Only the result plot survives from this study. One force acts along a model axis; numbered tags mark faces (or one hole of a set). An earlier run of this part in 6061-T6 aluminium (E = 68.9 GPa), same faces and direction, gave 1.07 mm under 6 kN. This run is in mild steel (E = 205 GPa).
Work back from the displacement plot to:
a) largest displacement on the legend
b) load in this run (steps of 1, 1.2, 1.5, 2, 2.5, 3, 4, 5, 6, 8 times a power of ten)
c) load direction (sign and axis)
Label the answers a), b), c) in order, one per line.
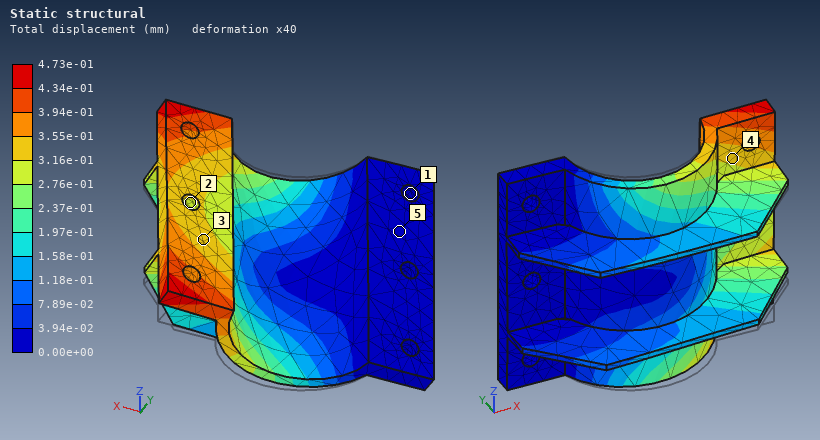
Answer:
a) 4.73e-01 mm
b) 8 kN
c) +Z
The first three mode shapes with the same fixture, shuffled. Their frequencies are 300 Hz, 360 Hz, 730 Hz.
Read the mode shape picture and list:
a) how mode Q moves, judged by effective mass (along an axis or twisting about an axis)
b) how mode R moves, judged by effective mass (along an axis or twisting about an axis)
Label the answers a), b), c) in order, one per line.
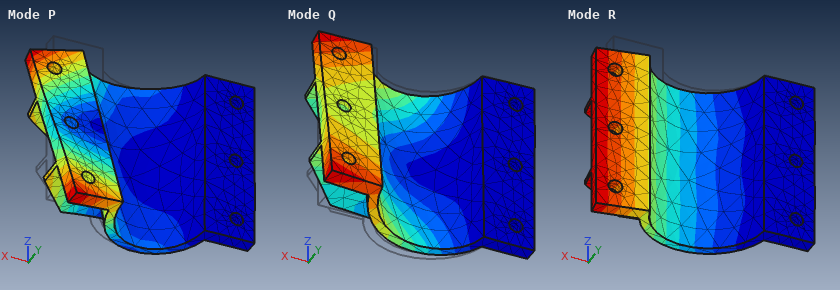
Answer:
a) along Z
b) along Y
